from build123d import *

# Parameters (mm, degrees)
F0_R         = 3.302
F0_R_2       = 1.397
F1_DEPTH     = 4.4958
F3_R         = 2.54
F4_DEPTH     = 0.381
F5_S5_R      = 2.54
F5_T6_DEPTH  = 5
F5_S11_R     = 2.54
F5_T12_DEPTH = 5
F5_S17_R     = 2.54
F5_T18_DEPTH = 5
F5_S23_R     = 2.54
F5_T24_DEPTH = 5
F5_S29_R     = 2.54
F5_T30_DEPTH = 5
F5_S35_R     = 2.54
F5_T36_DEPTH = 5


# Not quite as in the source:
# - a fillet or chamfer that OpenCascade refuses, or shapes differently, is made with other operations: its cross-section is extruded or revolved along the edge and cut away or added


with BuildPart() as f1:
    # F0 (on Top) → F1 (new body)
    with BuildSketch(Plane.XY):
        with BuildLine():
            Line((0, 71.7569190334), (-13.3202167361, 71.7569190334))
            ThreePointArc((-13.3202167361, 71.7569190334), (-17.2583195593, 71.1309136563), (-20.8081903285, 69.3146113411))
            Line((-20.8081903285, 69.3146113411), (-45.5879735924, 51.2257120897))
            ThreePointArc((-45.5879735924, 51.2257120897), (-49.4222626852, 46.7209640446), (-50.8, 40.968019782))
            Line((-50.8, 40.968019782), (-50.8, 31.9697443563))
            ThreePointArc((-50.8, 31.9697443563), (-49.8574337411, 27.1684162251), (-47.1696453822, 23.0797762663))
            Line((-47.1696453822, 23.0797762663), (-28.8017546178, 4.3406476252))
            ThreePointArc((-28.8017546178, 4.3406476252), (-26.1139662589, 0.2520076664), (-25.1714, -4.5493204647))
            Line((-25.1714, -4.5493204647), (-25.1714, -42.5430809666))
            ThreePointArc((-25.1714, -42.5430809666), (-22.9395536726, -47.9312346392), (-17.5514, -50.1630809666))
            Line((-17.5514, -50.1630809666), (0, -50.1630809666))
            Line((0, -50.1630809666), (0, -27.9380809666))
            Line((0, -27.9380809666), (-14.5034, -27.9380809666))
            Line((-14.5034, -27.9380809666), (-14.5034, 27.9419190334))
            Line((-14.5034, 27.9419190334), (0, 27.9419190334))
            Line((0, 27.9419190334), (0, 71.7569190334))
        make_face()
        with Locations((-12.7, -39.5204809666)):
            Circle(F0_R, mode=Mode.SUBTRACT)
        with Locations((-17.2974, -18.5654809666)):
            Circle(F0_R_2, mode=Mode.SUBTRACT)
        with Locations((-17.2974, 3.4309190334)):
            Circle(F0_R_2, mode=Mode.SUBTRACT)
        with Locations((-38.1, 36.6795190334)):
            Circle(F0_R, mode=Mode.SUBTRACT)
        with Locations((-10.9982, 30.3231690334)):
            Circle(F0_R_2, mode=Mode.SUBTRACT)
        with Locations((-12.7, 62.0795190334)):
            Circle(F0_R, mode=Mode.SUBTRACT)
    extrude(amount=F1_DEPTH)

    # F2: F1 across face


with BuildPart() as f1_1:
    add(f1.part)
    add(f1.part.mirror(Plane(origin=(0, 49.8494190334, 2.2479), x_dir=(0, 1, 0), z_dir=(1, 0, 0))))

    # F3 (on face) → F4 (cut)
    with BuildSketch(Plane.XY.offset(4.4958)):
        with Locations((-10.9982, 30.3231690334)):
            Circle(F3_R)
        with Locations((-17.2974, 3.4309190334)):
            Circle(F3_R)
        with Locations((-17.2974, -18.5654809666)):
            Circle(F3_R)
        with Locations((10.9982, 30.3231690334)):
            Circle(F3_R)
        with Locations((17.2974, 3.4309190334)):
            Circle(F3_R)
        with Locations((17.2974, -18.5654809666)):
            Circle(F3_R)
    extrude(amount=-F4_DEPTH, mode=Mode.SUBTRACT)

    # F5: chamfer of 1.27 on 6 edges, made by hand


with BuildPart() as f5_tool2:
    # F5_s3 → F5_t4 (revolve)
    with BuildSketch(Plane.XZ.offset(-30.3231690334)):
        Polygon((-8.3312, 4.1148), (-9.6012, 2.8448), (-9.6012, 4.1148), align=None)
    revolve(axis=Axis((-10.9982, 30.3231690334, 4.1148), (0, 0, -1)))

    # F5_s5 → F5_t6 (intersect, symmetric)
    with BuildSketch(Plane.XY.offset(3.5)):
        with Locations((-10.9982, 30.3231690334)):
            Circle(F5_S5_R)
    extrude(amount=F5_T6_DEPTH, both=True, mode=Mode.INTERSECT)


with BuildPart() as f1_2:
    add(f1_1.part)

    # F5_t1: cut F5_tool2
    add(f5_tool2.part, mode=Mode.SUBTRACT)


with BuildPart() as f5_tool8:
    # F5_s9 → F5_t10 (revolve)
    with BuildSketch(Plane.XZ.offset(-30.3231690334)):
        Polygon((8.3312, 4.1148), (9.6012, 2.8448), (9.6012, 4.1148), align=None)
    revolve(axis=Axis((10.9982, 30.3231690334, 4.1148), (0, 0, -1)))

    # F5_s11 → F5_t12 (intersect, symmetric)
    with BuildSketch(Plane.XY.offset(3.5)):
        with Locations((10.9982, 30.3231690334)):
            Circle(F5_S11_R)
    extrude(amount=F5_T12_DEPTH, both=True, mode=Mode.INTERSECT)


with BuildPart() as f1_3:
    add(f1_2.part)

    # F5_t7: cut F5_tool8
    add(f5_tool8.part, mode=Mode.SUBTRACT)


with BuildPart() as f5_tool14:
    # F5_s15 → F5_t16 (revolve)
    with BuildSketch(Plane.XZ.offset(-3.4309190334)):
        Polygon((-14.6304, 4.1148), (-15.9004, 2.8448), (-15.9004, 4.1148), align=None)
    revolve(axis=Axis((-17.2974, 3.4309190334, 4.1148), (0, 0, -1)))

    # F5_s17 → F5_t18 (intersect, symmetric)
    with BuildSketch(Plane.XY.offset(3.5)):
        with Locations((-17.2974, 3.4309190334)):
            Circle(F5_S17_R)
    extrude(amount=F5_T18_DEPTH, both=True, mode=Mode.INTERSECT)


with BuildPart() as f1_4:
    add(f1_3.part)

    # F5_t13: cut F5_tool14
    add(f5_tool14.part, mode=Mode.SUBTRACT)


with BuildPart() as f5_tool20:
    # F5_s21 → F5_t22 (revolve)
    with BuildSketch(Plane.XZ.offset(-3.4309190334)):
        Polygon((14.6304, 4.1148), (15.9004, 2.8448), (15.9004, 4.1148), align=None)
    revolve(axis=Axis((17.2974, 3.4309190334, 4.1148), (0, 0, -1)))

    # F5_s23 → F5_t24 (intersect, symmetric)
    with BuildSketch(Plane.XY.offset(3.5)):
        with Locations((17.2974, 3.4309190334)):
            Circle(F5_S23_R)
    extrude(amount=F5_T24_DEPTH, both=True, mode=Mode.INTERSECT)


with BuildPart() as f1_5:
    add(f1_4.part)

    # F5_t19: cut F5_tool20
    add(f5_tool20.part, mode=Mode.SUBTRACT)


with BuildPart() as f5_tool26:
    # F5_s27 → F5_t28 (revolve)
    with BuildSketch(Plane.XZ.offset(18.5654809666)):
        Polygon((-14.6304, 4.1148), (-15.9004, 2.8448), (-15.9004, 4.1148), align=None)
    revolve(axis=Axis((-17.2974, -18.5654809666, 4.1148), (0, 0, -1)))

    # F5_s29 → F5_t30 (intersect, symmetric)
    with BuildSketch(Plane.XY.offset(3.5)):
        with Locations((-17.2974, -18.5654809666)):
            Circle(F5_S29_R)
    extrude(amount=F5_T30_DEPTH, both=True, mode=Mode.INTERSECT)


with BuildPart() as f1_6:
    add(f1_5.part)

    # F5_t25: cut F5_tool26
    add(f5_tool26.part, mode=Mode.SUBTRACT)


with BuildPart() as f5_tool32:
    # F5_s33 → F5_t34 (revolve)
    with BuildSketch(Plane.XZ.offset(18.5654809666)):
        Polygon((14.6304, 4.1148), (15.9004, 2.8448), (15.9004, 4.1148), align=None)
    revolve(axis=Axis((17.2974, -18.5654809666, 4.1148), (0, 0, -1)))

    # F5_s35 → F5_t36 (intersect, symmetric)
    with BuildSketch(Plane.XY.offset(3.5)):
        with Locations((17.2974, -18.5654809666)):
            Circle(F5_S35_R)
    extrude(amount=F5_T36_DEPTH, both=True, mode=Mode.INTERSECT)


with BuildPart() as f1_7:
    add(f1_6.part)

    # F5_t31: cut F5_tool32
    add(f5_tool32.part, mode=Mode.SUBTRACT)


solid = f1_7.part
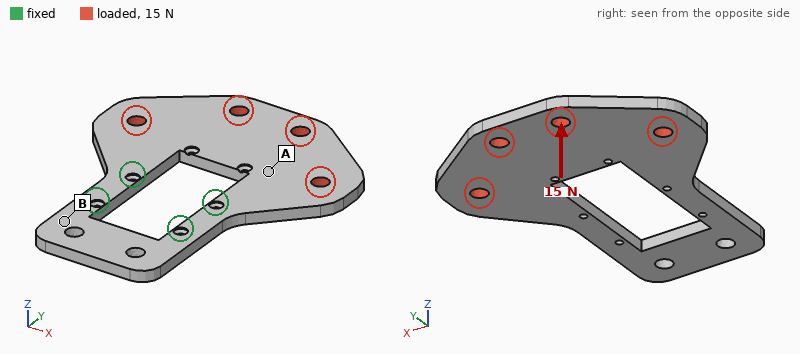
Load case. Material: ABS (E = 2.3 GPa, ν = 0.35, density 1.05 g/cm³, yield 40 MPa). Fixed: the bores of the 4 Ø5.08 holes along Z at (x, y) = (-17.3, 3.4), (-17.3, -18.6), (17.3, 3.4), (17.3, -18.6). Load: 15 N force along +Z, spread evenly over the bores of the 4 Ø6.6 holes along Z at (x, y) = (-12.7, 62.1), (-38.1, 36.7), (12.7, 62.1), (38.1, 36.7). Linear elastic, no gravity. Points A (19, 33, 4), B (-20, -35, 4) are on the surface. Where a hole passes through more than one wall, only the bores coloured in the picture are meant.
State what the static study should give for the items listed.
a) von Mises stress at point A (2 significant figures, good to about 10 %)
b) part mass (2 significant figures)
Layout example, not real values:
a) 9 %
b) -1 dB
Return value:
a) 1.4 MPa
b) 30 g
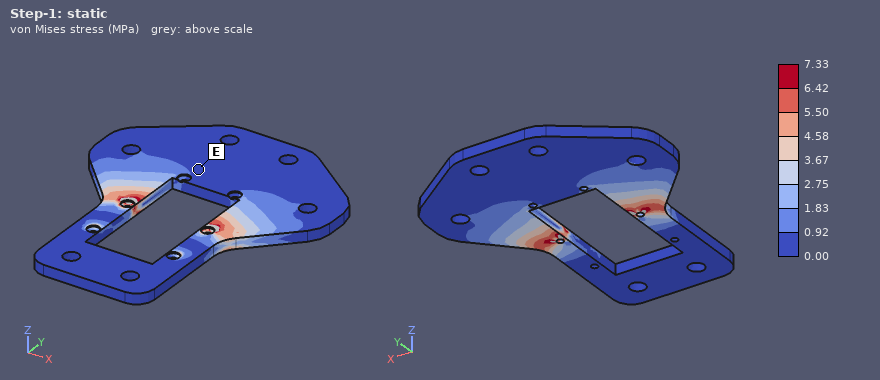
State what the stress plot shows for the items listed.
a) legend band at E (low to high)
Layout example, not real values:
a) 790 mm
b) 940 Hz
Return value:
a) 0.00 to 0.92 MPa
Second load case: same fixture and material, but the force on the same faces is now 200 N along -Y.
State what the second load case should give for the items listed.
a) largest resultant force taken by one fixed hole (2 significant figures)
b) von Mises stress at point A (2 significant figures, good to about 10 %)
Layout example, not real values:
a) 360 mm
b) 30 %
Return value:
a) 71 N
b) 1.1 MPa
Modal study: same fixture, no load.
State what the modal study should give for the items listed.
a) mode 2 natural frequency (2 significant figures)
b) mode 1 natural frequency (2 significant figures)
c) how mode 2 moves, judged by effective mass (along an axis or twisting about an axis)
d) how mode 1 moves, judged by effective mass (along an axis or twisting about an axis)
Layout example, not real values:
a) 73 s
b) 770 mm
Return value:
a) 330 Hz
b) 160 Hz
c) twisting about Y
d) along Z
